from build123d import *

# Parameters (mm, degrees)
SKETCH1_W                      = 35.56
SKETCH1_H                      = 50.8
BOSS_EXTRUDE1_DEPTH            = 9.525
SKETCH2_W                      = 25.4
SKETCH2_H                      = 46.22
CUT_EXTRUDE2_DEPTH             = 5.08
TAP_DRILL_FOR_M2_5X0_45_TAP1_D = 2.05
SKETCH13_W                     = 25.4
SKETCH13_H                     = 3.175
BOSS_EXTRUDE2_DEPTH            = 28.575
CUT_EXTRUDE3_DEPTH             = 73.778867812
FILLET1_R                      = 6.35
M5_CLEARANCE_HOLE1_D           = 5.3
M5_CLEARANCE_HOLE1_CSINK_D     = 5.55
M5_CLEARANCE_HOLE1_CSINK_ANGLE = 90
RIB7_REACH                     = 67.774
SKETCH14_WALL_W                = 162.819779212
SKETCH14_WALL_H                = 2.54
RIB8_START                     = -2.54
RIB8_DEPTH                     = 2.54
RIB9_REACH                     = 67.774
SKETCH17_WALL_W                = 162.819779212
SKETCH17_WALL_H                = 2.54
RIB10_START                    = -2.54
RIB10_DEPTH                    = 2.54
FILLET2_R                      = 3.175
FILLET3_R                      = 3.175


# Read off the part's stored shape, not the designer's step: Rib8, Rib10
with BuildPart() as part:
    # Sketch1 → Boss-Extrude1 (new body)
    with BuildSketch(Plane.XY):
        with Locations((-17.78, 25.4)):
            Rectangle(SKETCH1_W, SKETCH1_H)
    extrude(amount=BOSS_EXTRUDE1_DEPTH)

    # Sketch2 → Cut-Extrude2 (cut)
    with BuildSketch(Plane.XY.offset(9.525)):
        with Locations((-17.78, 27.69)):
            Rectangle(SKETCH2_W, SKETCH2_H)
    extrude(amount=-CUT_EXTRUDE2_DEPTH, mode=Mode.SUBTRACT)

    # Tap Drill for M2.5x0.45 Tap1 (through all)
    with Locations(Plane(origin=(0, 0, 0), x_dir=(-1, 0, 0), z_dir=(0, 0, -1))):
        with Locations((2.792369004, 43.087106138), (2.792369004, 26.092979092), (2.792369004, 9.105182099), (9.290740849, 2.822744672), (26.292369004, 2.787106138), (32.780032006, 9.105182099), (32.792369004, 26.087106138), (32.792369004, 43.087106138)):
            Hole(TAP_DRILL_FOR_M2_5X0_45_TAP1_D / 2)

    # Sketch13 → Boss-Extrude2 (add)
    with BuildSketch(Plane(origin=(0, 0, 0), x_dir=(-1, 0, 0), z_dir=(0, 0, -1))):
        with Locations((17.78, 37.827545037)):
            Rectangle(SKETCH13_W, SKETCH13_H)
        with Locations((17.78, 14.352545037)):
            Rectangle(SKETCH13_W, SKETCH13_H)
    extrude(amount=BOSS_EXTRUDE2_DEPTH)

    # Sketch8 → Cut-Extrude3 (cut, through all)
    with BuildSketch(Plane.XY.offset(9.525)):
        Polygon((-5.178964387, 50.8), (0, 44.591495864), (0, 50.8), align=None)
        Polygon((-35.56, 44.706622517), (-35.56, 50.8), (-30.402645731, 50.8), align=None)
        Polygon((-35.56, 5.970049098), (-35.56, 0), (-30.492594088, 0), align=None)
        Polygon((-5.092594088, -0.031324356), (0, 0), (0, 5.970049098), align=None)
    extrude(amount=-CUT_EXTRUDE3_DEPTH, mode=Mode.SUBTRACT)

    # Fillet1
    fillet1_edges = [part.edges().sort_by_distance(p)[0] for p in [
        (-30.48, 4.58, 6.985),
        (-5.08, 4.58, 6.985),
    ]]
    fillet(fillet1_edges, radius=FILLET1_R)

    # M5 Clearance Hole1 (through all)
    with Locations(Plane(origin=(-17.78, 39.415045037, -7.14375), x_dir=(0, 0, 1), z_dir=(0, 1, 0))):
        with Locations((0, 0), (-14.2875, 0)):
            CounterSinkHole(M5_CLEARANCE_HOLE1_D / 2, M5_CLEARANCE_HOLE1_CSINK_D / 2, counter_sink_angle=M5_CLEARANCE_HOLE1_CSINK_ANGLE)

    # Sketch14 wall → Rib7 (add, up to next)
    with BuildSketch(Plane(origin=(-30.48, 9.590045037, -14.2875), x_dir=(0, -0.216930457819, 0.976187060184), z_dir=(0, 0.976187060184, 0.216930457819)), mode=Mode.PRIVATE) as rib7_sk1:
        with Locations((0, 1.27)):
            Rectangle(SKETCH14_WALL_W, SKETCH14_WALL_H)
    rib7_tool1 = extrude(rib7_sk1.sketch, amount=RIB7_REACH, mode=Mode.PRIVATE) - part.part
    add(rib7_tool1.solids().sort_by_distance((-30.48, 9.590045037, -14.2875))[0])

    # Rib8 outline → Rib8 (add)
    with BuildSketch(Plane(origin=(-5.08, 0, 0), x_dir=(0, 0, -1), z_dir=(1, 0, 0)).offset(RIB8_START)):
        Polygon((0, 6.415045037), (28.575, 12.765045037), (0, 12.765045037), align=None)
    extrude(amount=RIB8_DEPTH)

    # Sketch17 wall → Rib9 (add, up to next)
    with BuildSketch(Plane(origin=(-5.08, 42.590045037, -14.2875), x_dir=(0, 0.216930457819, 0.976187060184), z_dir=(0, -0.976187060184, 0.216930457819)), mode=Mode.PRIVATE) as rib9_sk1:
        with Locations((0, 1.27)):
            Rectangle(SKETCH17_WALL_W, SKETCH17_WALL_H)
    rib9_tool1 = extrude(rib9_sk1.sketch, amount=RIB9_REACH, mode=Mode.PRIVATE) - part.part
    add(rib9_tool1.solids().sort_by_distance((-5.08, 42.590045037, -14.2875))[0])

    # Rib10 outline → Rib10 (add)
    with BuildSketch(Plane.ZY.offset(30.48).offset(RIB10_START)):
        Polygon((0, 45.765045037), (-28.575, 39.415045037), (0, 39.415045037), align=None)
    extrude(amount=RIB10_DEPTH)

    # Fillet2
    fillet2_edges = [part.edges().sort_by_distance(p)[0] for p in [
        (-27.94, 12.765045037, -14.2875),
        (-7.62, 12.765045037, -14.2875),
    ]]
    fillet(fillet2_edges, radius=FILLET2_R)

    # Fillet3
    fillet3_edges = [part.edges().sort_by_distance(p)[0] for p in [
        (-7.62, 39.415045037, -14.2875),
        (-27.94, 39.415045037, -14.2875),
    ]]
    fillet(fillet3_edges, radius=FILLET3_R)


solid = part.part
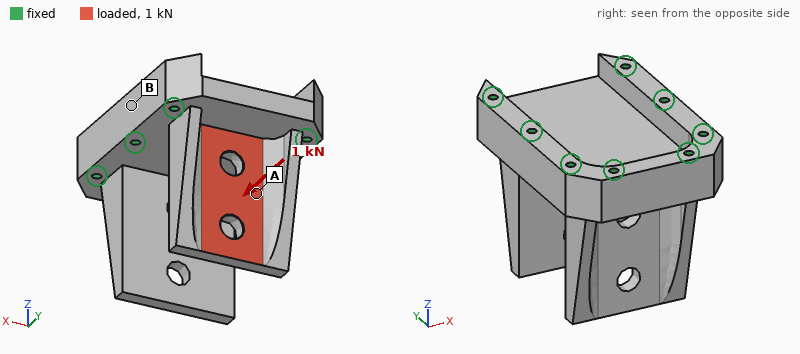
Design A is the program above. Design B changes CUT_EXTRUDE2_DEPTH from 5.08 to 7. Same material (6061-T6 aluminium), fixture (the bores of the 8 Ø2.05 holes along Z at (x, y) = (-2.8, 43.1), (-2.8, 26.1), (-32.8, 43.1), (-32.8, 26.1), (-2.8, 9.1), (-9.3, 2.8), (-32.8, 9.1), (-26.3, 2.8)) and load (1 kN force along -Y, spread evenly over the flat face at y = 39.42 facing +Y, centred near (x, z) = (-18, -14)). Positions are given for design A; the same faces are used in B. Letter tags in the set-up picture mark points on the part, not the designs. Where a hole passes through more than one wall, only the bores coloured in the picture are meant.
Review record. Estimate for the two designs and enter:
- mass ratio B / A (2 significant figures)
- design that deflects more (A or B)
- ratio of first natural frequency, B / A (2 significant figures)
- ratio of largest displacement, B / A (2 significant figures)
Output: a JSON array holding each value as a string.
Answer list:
["0.86", "B", "0.91", "1.2"]
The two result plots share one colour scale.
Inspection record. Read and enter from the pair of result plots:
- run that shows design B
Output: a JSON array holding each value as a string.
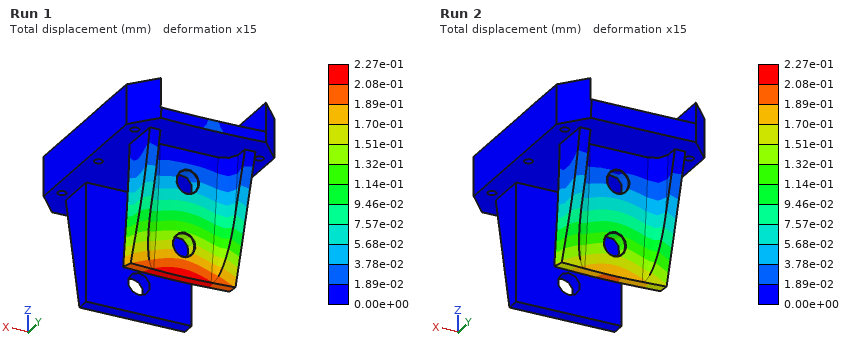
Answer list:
["Run 1"]
